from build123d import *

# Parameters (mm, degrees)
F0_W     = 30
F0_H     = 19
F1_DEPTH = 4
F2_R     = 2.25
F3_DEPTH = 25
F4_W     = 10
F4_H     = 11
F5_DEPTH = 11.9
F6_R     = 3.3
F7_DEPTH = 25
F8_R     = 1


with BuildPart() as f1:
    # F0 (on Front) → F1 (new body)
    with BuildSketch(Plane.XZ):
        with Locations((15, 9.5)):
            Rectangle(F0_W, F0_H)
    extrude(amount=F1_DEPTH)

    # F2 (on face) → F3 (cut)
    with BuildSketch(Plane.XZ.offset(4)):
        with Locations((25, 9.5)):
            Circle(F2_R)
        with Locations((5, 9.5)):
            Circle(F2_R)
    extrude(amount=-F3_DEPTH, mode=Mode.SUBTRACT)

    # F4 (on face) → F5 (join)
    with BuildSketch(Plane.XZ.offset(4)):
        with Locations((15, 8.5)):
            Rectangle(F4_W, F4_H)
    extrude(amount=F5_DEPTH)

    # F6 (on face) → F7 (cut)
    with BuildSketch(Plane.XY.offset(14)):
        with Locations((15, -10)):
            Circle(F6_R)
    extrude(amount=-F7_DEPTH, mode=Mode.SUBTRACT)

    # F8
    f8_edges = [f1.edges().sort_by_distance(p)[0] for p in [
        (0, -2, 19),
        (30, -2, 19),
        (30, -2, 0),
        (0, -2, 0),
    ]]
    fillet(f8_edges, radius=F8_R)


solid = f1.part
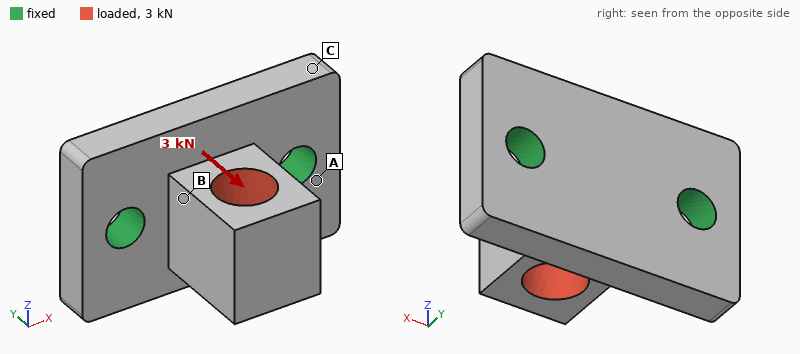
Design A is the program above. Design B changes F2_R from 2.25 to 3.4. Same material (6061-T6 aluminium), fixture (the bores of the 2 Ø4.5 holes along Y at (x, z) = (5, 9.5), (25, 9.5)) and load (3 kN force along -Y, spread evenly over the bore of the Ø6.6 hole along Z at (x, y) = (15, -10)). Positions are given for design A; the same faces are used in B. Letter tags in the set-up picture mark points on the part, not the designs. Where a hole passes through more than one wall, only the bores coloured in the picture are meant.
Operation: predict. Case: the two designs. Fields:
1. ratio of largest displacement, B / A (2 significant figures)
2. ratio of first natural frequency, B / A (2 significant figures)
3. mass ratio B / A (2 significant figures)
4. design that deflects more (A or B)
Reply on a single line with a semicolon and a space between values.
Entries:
0.72; 1.2; 0.95; A
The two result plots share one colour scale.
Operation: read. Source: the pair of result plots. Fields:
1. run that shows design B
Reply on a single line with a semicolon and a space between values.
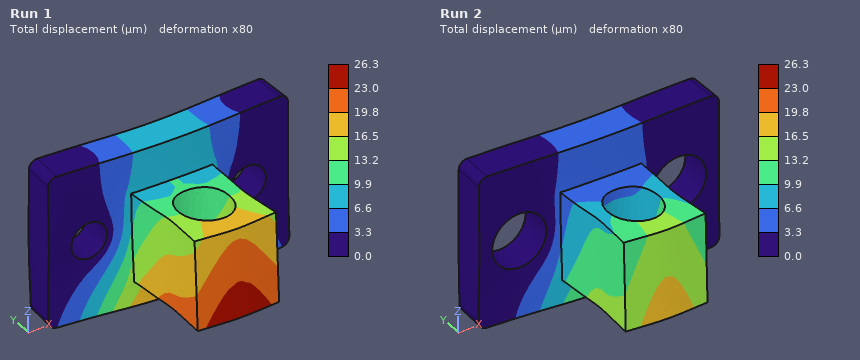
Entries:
Run 2
